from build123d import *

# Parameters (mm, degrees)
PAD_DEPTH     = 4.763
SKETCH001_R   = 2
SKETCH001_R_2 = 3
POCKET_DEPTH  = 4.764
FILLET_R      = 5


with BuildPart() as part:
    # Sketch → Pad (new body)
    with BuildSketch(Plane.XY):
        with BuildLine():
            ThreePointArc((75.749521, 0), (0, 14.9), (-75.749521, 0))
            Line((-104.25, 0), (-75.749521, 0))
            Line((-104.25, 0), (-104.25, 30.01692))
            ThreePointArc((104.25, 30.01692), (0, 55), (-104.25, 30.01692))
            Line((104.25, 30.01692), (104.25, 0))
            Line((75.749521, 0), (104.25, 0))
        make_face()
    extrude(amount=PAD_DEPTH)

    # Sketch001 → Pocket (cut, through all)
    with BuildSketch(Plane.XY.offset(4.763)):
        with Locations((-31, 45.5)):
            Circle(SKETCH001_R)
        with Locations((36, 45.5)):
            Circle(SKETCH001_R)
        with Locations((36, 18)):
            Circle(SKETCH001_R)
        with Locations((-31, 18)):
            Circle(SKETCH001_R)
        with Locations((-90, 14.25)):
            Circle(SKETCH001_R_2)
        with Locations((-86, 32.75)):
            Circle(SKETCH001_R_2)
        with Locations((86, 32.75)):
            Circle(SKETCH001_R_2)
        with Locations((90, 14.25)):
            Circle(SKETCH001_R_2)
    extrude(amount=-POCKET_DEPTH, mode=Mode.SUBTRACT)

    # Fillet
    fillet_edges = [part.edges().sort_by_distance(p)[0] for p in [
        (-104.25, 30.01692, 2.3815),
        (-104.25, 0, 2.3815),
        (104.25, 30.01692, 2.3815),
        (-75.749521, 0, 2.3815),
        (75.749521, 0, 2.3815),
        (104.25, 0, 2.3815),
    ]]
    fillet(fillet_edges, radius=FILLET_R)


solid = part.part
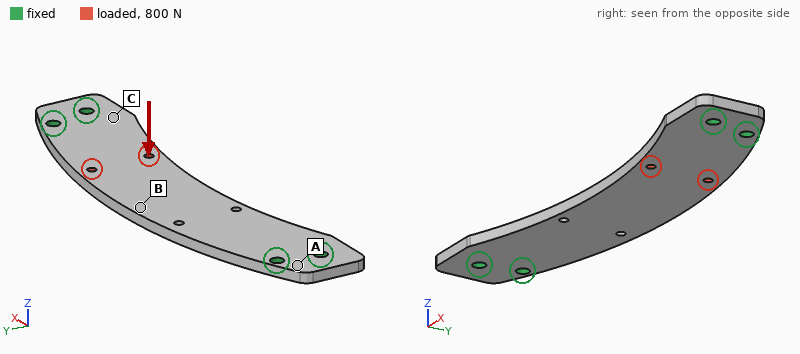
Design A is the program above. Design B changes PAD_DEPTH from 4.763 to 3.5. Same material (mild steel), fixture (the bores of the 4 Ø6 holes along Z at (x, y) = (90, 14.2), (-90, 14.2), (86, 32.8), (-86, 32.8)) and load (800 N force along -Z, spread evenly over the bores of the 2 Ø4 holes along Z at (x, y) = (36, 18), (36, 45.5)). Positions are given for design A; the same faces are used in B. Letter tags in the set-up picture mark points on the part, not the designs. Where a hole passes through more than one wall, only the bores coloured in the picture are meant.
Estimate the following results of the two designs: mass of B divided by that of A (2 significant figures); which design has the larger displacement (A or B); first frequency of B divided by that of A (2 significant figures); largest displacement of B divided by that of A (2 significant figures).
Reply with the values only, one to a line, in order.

0.73
B
0.74
2.5
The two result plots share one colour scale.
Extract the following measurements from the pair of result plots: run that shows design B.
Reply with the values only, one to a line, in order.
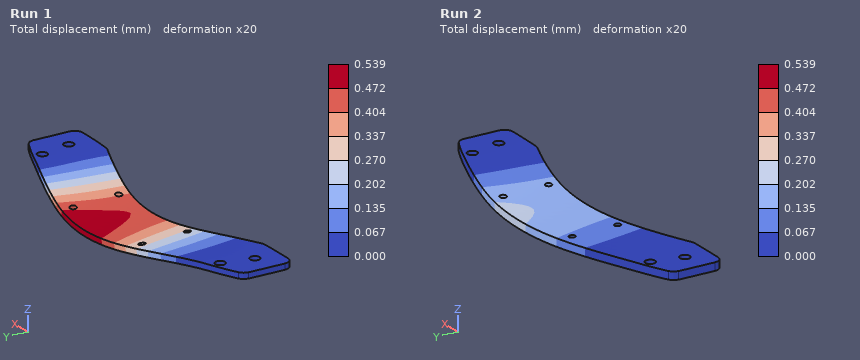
Run 1
